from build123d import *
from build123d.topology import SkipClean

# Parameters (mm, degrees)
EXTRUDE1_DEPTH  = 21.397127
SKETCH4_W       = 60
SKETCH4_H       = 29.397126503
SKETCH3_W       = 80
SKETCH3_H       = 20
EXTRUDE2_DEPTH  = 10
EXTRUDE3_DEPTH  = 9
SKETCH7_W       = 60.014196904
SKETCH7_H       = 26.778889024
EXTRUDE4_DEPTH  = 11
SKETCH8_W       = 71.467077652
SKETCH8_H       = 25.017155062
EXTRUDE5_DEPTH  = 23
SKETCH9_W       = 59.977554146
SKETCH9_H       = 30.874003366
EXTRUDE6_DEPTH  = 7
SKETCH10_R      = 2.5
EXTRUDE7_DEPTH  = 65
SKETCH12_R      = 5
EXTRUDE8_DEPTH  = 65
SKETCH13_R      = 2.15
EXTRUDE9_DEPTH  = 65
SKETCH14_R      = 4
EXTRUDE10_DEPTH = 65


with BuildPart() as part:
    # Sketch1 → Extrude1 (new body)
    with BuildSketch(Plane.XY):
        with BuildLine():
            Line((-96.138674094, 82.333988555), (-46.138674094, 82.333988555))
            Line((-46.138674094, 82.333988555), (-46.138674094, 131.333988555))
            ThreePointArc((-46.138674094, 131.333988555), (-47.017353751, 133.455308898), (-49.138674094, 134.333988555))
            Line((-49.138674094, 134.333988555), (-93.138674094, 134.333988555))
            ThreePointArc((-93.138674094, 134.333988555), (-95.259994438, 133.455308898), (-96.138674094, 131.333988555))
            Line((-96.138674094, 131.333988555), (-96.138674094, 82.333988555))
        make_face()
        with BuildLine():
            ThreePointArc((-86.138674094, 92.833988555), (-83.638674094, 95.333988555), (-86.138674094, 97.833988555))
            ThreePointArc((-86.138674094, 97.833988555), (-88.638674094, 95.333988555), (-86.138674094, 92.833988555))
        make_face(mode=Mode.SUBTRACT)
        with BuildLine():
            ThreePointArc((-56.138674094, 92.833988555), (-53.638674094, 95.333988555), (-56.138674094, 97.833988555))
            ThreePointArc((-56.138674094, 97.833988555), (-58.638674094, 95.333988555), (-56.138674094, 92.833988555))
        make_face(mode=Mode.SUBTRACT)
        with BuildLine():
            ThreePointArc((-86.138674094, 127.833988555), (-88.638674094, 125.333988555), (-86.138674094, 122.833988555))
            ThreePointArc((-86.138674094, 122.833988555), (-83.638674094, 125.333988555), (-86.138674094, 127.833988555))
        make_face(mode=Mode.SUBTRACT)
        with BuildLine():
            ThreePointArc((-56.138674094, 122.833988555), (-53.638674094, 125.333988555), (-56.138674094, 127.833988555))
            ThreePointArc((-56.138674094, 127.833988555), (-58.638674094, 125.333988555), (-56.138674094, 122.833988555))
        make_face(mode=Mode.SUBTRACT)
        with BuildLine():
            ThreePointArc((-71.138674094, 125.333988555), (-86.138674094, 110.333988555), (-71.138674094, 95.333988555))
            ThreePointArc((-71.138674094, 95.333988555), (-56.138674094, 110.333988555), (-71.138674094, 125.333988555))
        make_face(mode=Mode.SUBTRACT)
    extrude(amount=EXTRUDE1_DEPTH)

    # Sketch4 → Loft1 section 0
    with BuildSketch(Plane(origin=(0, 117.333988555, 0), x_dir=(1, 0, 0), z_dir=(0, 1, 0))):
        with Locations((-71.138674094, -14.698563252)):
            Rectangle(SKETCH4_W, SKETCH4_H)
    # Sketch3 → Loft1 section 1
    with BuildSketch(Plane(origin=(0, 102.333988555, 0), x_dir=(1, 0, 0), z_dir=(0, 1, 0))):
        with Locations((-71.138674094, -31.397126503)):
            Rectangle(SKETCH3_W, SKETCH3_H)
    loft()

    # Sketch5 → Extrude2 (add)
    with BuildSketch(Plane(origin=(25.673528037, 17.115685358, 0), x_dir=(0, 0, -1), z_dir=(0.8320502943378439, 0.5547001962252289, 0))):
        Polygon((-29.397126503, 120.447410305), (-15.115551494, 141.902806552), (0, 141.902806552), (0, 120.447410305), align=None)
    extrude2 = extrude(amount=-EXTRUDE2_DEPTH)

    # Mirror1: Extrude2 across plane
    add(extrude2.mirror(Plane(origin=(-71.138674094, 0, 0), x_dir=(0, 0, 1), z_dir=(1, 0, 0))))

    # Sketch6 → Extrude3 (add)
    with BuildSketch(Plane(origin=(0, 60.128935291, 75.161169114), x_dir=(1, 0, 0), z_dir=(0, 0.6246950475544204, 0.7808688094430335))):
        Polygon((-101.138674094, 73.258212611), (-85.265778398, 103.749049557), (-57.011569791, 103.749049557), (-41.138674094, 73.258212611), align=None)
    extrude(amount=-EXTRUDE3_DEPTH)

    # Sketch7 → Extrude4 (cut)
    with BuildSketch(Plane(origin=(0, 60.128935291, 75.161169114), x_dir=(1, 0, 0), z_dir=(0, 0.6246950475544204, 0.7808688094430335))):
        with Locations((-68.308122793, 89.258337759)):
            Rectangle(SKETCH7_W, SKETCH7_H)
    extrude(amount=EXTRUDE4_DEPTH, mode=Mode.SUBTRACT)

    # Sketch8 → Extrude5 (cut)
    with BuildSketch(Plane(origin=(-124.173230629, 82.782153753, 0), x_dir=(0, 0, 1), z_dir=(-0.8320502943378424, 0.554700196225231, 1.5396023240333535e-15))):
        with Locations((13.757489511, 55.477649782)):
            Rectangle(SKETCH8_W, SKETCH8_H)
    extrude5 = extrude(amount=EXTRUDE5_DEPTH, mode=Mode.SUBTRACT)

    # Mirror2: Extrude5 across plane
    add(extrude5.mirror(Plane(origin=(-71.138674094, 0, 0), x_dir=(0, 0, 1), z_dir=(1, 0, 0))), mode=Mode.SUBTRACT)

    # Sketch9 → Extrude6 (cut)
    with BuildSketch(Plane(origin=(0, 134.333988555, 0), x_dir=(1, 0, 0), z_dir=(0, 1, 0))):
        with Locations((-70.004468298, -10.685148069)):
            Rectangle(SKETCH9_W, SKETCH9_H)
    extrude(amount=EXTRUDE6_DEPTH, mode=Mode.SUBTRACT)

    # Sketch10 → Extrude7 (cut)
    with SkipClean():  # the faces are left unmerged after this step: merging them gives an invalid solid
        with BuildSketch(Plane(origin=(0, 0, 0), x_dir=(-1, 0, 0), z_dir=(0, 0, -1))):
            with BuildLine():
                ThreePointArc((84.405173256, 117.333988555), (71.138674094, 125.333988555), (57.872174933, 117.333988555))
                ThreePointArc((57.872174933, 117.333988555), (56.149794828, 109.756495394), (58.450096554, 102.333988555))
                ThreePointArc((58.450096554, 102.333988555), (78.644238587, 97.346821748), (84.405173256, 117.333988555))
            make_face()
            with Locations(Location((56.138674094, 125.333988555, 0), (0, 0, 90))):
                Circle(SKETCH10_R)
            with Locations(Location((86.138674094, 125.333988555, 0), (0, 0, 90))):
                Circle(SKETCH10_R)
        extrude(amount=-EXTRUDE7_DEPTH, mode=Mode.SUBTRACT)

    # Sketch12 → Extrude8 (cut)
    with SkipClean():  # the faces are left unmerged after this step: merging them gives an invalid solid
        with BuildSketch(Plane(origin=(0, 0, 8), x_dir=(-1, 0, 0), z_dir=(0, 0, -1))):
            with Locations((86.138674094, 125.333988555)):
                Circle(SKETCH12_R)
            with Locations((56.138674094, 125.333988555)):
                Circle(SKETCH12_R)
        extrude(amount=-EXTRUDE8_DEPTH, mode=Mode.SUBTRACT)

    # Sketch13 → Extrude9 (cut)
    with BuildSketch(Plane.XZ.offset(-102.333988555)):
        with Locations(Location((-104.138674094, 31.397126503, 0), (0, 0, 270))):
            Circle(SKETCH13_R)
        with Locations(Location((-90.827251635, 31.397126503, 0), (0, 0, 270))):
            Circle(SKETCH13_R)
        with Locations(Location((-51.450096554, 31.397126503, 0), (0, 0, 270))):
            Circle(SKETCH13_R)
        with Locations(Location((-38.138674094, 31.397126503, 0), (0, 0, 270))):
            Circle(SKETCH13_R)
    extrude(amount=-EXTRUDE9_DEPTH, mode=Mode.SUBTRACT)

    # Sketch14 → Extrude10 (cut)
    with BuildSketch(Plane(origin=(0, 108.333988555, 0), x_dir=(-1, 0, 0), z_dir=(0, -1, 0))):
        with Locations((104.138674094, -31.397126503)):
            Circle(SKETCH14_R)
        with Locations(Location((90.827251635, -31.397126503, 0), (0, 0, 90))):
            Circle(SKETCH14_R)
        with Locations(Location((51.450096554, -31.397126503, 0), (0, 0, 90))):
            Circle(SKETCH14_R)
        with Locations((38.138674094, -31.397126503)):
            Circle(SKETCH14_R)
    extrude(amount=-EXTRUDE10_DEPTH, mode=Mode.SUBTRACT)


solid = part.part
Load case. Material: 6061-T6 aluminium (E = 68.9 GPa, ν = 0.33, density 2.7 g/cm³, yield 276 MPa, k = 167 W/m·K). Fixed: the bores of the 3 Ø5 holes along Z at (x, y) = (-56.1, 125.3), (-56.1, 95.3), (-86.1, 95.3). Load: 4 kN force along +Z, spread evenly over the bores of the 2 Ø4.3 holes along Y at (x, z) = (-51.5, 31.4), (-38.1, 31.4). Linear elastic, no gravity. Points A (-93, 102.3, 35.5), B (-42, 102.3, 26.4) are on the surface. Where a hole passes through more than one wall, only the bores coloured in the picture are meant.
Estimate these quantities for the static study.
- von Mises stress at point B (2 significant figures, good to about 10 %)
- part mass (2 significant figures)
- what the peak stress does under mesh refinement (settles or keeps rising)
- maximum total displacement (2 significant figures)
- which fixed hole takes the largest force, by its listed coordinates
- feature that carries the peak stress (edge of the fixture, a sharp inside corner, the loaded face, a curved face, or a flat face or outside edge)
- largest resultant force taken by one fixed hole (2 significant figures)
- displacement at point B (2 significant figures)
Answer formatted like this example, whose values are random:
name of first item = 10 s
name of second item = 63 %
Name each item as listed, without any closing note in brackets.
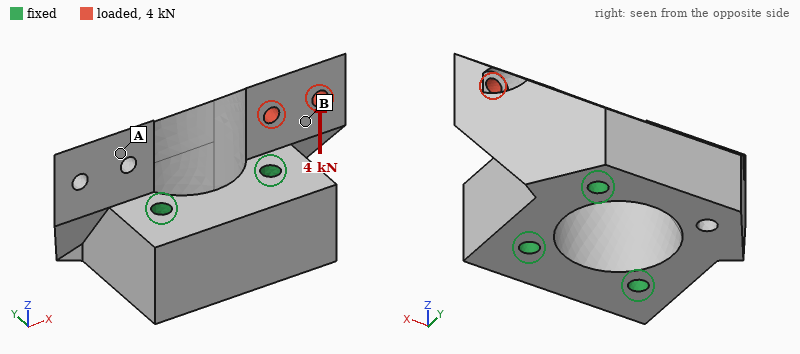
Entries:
von Mises stress at point B = 30 MPa
part mass = 130 g
what the peak stress does under mesh refinement = keeps rising
maximum total displacement = 62 µm
which fixed hole takes the largest force, by its listed coordinates = (-56.1, 95.3)
feature that carries the peak stress = edge of the fixture
largest resultant force taken by one fixed hole = 3.2 kN
displacement at point B = 31 µm
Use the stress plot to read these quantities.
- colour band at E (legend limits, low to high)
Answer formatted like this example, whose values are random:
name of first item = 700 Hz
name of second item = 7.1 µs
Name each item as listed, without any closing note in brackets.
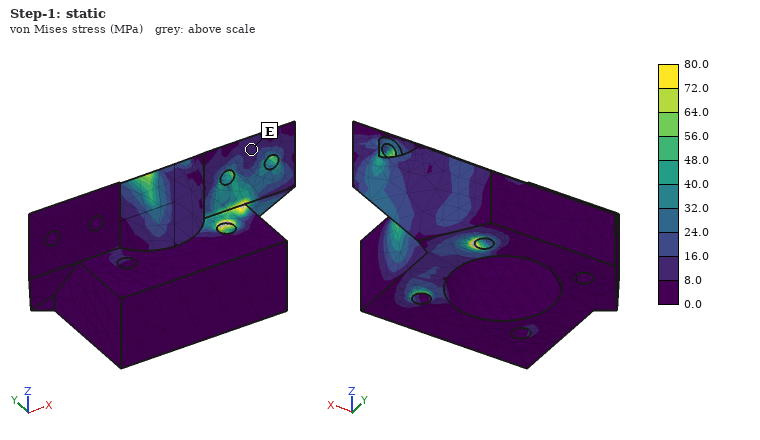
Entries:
colour band at E = 8.0 to 16.0 MPa
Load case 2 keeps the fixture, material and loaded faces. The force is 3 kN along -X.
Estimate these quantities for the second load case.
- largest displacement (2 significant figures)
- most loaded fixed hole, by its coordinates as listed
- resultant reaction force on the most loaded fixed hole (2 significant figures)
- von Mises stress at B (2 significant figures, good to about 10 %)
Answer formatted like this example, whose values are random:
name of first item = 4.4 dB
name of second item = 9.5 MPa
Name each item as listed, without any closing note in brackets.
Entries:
largest displacement = 91 µm
most loaded fixed hole, by its coordinates as listed = (-56.1, 95.3)
resultant reaction force on the most loaded fixed hole = 2.9 kN
von Mises stress at B = 36 MPa
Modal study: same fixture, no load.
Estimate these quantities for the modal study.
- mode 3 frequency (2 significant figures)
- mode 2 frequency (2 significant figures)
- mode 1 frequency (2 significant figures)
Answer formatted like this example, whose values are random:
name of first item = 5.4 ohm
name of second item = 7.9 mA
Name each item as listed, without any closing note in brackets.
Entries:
mode 3 frequency = 12 kHz
mode 2 frequency = 10 kHz
mode 1 frequency = 8800 Hz
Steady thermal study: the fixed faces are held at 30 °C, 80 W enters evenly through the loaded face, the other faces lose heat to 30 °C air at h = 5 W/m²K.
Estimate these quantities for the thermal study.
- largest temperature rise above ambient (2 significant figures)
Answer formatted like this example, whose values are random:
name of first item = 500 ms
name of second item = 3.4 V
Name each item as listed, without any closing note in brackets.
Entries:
largest temperature rise above ambient = 58 K
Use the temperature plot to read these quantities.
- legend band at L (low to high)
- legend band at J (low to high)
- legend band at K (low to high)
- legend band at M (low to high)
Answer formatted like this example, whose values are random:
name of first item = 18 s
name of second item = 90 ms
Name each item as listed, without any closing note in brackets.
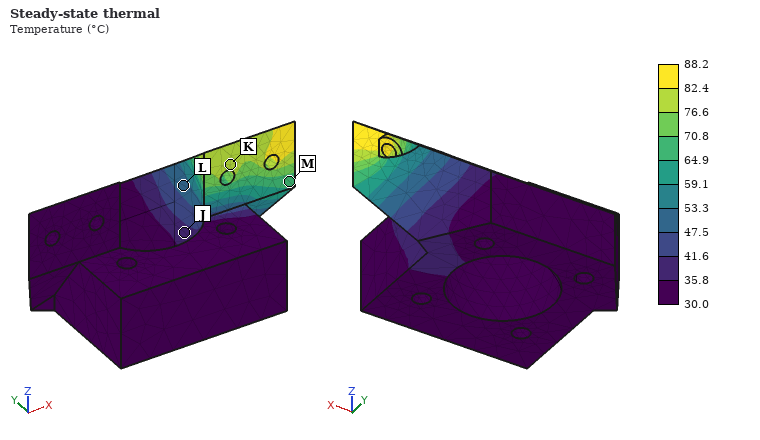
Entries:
legend band at L = 47.5 to 53.3 °C
legend band at J = 35.8 to 41.6 °C
legend band at K = 76.6 to 82.4 °C
legend band at M = 64.9 to 70.8 °C
